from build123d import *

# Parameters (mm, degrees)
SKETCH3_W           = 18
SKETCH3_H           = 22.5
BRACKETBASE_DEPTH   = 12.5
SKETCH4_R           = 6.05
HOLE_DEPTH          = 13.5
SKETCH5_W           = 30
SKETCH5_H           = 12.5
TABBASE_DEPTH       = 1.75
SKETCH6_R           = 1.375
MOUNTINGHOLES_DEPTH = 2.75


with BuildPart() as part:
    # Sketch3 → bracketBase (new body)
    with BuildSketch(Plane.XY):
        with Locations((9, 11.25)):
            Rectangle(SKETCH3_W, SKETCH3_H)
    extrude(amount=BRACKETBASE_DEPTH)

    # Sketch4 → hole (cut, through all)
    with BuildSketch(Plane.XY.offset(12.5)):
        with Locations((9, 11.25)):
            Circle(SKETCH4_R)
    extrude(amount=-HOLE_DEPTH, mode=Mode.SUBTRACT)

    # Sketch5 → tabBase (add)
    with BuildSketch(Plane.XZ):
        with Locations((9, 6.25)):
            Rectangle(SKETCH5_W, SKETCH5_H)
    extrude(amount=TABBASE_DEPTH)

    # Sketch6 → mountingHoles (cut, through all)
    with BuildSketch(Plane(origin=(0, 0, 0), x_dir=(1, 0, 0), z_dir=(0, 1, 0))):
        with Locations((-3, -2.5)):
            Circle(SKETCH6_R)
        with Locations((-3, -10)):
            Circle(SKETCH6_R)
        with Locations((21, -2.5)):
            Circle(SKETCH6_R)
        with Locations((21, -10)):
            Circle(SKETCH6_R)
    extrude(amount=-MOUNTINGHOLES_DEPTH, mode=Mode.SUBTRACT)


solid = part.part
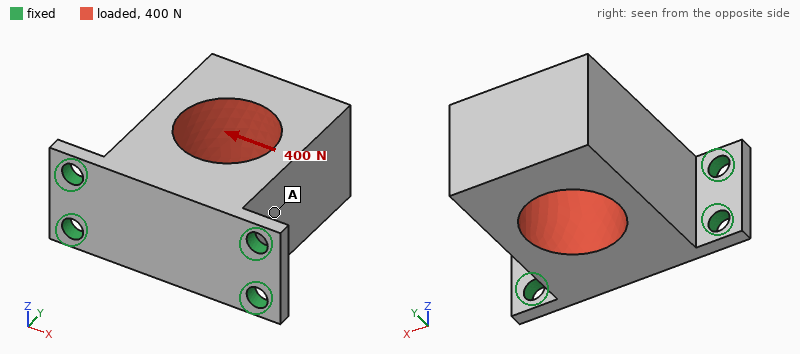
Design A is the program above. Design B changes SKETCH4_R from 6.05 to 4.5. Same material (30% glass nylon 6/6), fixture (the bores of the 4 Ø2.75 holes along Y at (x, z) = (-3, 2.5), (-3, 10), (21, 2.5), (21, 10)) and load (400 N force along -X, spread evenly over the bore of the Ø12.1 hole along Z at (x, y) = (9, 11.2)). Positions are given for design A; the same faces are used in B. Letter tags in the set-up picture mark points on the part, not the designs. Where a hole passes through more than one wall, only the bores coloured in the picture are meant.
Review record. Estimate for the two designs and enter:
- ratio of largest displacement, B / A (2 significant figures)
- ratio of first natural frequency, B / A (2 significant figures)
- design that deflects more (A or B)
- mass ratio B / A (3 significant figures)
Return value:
0.78
0.95
A
1.15
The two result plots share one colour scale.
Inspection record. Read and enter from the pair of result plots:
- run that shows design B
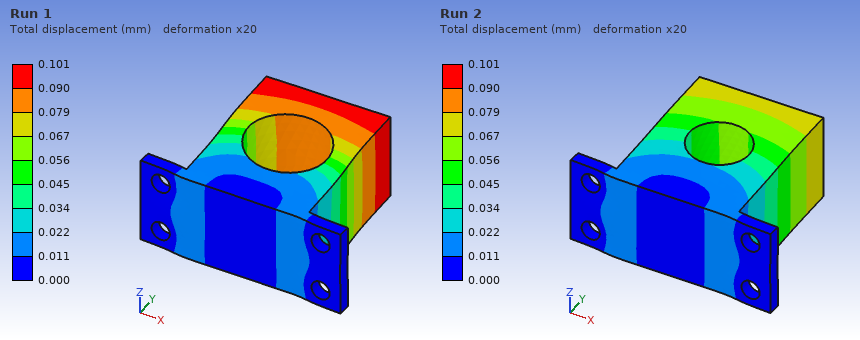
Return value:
Run 2
